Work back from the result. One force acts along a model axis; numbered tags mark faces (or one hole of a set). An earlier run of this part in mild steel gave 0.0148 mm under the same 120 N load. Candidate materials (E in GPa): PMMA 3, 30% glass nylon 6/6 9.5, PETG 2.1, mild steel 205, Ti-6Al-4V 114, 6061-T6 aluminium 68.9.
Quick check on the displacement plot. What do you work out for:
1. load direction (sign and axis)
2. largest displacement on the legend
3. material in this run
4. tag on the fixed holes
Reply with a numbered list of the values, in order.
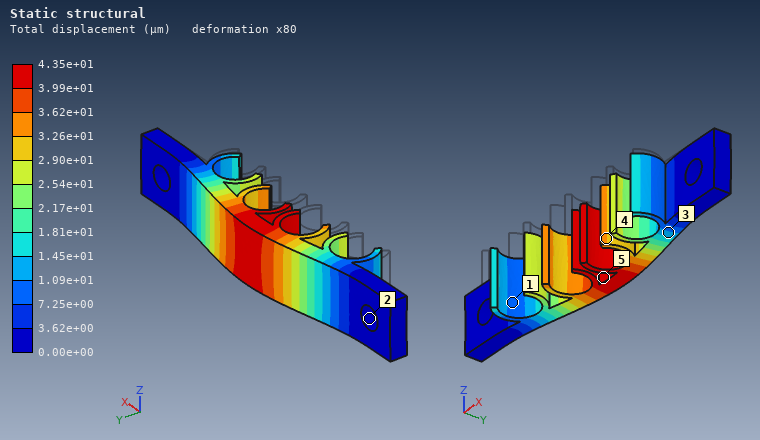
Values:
1. +Y
2. 4.35e+01 µm
3. 6061-T6 aluminium
4. 2
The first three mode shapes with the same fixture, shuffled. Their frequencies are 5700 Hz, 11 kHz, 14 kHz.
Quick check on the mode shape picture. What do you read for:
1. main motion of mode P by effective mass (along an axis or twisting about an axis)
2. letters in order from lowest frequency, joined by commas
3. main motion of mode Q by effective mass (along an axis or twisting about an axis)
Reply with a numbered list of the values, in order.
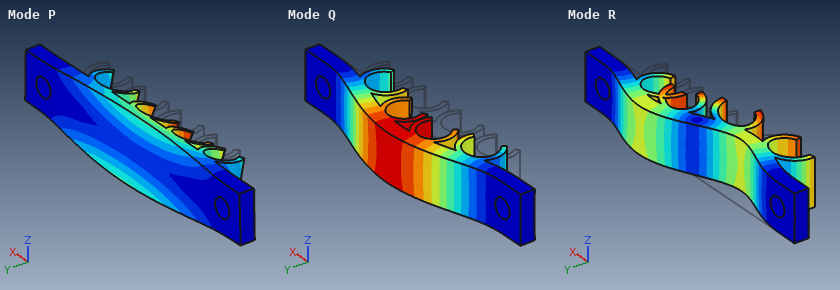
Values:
1. along Z
2. Q, P, R
3. along Y
